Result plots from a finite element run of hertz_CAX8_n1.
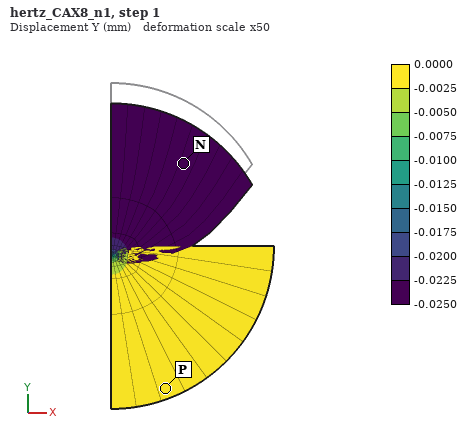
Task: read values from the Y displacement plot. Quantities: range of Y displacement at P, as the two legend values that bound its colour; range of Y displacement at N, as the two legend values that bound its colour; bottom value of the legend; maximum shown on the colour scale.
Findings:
-0.0025 to 0.0000 mm
-0.0250 to -0.0225 mm
-0.0250 mm
0.0000 mm
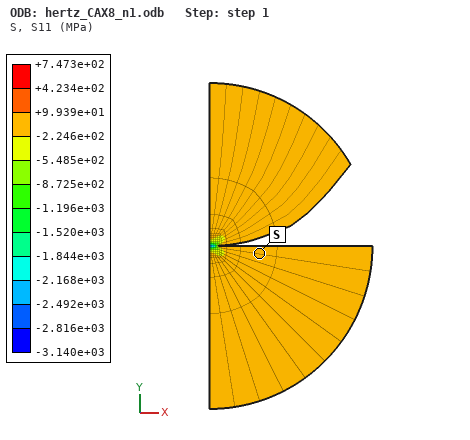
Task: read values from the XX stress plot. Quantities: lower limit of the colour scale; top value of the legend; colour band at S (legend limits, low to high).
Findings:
-3.140e+03 MPa
+7.473e+02 MPa
-2.246e+02 to +9.939e+01 MPa
